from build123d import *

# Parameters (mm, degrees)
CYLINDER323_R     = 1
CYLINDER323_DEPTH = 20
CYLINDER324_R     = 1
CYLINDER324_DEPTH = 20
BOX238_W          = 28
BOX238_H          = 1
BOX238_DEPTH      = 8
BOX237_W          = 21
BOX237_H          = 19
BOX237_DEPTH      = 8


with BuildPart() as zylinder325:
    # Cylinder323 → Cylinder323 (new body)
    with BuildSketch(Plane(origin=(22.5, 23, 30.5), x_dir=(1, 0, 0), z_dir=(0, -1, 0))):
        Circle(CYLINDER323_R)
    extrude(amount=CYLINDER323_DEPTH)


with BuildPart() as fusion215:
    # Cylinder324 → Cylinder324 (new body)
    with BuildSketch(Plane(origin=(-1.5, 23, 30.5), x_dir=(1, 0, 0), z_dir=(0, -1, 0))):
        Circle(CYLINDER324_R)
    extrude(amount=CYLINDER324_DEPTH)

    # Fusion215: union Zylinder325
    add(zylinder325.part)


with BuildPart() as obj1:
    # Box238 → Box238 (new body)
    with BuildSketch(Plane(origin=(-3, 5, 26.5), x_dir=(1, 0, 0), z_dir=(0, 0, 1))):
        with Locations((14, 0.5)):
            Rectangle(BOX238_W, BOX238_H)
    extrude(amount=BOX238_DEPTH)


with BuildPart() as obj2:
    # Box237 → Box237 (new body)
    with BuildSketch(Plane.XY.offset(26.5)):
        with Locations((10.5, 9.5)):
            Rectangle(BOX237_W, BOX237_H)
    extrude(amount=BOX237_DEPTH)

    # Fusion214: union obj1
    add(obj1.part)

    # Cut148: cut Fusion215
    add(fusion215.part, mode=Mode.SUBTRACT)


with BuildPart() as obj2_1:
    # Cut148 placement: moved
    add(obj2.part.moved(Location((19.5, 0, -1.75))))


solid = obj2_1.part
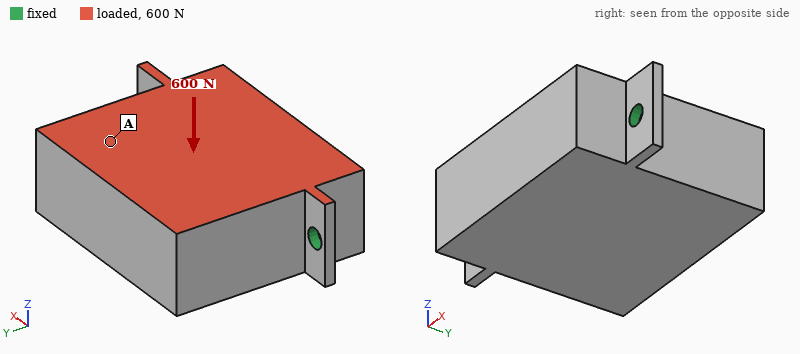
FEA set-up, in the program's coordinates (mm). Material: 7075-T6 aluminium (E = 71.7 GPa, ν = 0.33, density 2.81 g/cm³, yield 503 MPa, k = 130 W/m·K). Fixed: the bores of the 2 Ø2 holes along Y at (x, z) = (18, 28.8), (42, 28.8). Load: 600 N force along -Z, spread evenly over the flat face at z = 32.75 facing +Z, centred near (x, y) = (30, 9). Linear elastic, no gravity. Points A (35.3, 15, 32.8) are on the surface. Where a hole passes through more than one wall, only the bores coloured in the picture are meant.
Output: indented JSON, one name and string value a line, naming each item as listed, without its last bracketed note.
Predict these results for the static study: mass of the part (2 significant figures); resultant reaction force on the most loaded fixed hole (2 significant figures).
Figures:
{
  "mass of the part": "9.1 g",
  "resultant reaction force on the most loaded fixed hole": "300 N"
}
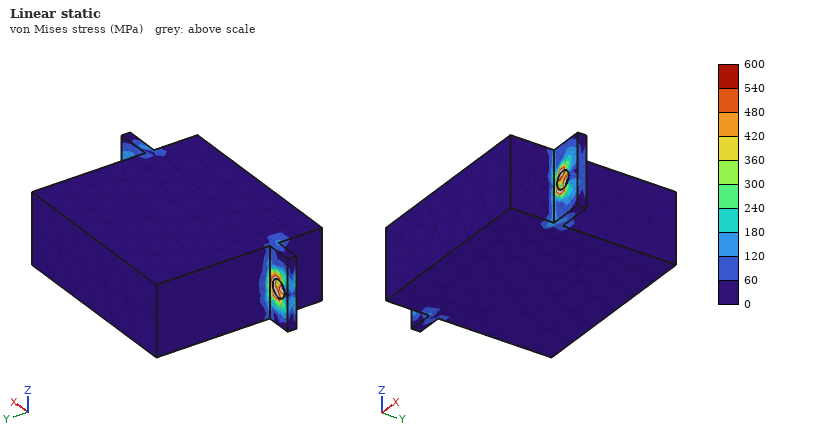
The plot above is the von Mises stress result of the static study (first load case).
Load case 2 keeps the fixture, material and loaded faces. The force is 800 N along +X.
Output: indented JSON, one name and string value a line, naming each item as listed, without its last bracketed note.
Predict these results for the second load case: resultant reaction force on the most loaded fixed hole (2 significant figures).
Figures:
{
  "resultant reaction force on the most loaded fixed hole": "450 N"
}
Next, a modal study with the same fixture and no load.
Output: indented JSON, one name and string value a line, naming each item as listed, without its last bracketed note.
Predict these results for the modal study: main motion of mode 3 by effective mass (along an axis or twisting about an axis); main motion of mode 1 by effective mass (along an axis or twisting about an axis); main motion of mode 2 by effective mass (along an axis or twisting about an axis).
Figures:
{
  "main motion of mode 3 by effective mass": "along X",
  "main motion of mode 1 by effective mass": "along Z",
  "main motion of mode 2 by effective mass": "along Y"
}
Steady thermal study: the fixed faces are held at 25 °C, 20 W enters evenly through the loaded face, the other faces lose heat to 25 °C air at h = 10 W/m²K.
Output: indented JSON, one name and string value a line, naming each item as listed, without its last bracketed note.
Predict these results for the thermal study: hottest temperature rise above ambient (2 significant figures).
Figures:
{
  "hottest temperature rise above ambient": "28 K"
}
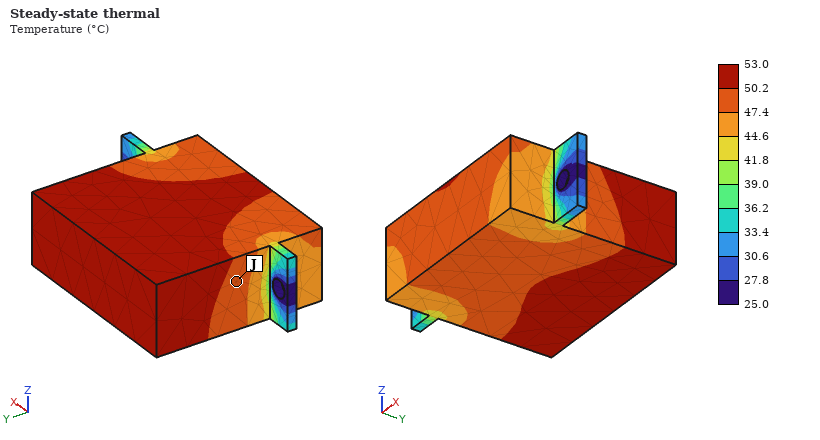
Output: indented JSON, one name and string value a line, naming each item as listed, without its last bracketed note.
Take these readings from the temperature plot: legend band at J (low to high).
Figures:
{
  "legend band at J": "47.4 to 50.2 °C"
}
